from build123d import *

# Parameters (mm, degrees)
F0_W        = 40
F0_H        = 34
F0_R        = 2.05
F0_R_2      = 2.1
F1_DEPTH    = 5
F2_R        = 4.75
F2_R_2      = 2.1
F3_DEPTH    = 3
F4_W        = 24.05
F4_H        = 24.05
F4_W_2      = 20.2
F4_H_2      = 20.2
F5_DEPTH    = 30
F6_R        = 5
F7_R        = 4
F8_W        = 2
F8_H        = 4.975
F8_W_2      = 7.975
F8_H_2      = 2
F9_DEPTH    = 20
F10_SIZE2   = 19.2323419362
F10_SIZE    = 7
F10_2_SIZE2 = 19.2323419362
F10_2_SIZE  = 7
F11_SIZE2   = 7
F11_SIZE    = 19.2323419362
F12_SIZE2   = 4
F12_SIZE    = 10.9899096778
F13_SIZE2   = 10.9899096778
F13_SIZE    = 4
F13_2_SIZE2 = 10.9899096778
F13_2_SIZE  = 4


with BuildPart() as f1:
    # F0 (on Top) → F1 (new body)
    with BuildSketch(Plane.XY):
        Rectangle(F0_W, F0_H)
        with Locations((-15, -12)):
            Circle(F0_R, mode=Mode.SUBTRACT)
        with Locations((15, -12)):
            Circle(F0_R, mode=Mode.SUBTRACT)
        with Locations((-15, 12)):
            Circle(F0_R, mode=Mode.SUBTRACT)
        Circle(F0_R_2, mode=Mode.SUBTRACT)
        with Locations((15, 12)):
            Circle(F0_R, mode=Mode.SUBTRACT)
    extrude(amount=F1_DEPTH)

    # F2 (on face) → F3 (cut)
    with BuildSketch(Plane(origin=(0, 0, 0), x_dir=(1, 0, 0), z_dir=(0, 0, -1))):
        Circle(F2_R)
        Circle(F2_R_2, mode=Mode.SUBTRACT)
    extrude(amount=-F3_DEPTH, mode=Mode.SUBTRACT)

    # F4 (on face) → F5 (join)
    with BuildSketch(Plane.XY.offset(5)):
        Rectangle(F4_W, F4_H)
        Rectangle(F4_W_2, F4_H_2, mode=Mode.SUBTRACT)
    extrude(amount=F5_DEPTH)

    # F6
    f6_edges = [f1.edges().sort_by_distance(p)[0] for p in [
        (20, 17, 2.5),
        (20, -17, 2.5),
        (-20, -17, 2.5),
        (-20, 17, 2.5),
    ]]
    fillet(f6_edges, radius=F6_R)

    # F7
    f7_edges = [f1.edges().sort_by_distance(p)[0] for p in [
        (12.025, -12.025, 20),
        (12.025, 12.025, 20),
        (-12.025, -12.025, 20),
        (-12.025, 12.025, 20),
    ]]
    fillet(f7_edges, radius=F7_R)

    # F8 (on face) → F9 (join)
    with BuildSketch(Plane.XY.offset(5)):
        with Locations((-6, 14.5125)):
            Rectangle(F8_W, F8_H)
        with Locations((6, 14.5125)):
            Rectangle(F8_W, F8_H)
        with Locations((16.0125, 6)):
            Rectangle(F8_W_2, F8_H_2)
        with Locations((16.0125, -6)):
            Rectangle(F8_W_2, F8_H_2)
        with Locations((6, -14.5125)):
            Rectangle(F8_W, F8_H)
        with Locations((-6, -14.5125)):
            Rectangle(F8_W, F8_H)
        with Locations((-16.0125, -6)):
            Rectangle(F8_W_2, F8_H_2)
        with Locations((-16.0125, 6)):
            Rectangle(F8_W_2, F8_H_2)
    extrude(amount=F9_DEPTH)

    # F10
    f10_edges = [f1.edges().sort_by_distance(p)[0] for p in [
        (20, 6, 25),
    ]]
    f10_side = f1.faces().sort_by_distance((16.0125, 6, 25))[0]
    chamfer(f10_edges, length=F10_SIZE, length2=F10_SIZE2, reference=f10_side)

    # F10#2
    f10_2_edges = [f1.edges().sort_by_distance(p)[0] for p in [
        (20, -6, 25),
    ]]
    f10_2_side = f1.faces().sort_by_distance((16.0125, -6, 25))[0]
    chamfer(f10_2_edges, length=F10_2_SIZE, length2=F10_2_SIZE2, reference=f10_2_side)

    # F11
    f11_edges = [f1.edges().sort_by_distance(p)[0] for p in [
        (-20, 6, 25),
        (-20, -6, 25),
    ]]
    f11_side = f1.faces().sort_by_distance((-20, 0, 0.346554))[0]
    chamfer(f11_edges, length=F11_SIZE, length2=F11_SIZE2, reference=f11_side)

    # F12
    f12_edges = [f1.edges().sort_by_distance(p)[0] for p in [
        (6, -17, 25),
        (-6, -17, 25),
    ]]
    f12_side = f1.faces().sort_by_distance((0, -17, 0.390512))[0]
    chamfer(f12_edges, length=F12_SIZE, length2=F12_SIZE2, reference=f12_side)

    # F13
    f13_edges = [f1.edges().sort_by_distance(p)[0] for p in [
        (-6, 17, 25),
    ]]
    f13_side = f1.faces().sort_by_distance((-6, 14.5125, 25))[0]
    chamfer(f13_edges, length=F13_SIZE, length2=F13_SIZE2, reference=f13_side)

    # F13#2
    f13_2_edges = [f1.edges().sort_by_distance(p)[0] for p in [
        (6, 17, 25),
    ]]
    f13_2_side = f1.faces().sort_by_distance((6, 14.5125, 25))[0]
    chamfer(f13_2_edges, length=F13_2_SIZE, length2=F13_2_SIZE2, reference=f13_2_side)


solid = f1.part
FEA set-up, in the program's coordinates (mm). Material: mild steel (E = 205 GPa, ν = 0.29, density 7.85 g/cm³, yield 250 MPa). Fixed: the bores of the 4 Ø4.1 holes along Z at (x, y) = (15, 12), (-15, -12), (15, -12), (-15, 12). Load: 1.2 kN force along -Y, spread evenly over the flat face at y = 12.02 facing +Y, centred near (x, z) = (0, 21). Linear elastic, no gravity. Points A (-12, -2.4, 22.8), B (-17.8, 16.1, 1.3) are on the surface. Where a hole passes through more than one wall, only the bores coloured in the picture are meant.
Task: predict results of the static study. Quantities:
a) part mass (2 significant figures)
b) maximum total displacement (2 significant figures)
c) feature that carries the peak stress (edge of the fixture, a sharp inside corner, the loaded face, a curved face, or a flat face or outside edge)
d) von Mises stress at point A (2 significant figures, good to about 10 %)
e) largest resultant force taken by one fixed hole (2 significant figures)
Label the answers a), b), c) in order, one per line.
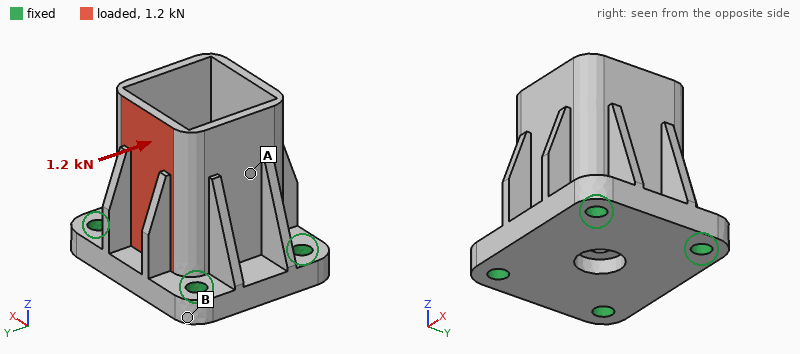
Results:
a) 96 g
b) 41 µm
c) the loaded face
d) 20 MPa
e) 570 N
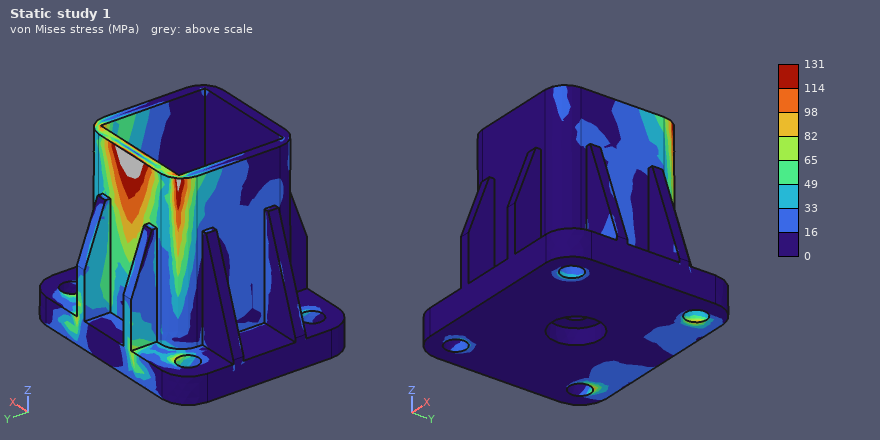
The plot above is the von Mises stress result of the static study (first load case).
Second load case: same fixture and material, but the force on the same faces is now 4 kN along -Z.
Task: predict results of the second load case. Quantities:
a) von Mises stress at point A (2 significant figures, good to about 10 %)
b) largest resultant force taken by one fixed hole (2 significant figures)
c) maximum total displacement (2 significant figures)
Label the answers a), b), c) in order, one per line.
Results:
a) 13 MPa
b) 2.1 kN
c) 30 µm
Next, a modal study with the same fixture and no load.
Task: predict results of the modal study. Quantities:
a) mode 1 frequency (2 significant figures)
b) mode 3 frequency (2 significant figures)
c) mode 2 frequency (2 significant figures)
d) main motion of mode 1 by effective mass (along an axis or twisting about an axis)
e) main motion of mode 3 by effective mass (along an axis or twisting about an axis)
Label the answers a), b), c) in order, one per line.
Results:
a) 11 kHz
b) 13 kHz
c) 11 kHz
d) along Y
e) along X
